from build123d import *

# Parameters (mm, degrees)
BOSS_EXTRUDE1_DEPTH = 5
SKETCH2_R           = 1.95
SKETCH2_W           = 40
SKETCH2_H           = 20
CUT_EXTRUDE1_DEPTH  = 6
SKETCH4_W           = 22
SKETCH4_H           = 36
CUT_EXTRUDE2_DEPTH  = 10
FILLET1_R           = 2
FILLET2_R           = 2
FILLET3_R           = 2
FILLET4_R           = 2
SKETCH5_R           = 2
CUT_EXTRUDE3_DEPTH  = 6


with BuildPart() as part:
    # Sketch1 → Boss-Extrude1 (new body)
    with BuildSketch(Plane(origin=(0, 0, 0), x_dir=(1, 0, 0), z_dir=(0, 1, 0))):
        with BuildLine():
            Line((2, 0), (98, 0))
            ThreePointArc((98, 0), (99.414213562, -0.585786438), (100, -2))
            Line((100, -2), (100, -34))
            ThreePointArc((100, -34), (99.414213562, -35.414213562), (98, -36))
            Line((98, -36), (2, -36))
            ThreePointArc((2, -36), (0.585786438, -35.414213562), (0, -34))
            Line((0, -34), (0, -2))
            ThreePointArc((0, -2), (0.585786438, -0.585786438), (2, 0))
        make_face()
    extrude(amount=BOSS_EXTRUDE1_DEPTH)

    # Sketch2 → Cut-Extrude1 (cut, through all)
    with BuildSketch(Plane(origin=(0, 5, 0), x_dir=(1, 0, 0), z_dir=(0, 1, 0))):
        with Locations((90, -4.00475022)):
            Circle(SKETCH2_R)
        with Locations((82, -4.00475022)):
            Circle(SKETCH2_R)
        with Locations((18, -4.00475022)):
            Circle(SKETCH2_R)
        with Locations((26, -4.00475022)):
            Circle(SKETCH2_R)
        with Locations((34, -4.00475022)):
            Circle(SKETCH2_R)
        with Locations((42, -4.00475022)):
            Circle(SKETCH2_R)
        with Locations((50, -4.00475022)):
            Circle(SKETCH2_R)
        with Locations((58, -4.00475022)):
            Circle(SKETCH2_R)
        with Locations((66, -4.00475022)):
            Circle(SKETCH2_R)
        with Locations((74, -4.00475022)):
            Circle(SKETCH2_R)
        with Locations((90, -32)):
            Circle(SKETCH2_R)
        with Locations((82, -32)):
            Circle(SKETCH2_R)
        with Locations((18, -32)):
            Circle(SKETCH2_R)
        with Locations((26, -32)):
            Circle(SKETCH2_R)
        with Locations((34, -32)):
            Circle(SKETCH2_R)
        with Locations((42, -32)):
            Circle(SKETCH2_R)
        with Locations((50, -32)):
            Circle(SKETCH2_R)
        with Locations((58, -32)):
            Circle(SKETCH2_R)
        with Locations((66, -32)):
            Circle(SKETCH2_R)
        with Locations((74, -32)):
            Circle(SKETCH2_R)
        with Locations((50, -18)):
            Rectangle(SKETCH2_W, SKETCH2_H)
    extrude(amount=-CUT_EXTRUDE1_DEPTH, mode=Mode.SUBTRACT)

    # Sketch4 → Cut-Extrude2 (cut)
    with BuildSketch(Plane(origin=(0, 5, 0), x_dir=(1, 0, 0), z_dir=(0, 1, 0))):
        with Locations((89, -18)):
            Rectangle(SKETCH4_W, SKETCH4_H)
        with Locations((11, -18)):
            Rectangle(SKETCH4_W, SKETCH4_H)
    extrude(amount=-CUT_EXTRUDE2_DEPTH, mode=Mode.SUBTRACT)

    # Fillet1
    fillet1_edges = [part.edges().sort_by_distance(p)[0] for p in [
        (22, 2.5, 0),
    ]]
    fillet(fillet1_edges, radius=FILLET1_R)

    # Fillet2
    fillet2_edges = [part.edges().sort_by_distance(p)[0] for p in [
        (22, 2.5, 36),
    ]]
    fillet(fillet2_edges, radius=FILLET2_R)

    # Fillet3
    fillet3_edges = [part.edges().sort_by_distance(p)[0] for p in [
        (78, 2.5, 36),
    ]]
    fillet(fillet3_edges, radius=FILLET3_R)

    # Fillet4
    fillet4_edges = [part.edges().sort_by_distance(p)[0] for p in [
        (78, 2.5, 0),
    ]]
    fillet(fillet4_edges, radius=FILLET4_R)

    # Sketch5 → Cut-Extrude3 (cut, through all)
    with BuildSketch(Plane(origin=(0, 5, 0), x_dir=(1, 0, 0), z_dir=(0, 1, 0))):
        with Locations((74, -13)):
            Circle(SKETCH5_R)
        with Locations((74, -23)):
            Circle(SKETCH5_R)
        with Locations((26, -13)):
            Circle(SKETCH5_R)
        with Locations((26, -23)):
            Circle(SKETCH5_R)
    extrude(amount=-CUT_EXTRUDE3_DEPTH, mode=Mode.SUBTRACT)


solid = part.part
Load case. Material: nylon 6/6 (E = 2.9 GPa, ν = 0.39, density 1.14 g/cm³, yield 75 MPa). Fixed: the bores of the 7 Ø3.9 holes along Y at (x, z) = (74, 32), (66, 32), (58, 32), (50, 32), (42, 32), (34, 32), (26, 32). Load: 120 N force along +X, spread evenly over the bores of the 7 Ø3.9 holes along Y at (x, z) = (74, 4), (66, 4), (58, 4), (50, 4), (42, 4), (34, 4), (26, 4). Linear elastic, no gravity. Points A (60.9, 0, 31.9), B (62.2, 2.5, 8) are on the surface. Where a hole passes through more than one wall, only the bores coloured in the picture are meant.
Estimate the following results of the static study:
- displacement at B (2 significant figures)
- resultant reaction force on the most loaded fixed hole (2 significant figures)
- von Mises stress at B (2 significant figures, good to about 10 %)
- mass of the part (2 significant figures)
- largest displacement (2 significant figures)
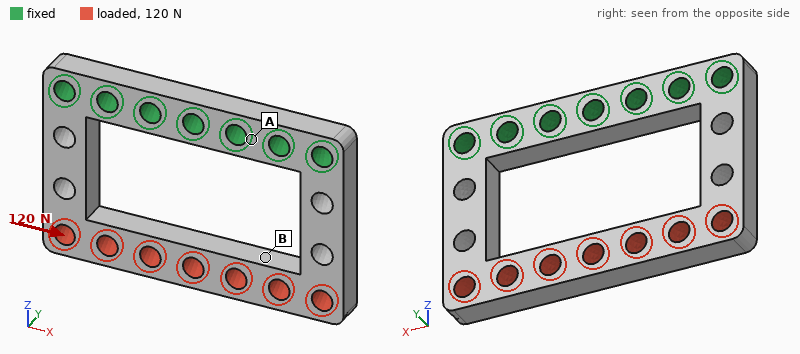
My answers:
0.36 mm
100 N
7.0 MPa
5.7 g
0.39 mm
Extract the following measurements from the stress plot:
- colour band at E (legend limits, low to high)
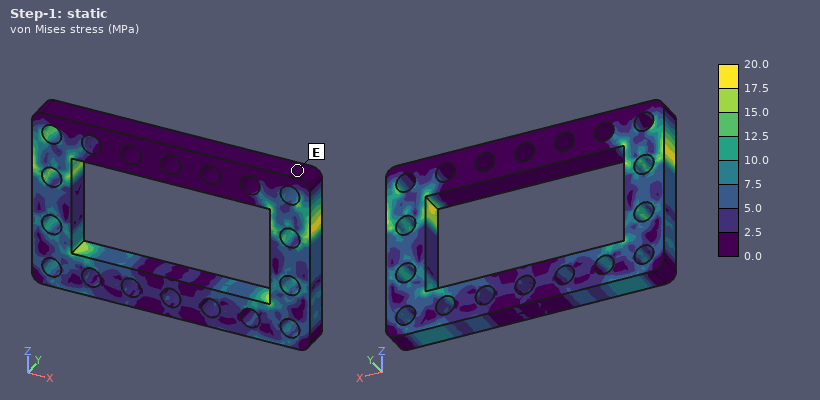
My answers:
0.0 to 2.5 MPa
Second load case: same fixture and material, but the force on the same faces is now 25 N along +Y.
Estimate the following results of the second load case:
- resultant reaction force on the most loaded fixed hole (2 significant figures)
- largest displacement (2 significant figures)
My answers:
11 N
0.67 mm
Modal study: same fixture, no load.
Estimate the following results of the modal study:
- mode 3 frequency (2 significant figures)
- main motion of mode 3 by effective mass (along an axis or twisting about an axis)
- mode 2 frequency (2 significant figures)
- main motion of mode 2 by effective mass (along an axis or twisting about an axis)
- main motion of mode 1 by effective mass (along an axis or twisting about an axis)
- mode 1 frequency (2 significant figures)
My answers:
1800 Hz
along X
1400 Hz
twisting about Z
along Y
730 Hz
